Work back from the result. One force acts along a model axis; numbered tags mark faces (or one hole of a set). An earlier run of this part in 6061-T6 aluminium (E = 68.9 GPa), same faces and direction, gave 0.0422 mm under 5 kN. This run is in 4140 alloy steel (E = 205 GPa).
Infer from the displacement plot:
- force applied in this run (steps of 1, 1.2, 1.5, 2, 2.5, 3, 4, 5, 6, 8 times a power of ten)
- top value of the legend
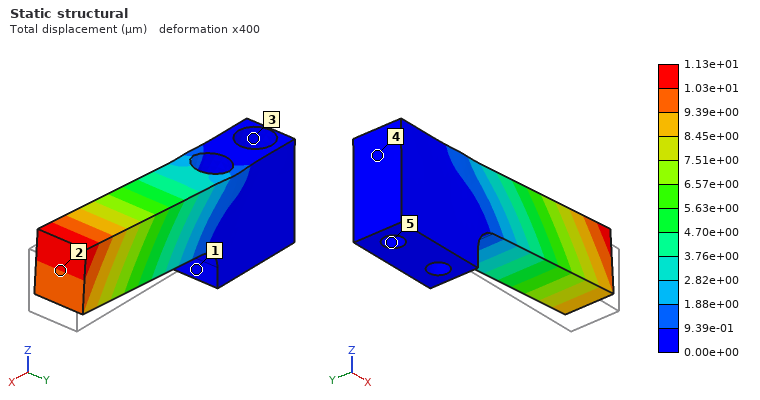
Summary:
4 kN
1.13e+01 µm
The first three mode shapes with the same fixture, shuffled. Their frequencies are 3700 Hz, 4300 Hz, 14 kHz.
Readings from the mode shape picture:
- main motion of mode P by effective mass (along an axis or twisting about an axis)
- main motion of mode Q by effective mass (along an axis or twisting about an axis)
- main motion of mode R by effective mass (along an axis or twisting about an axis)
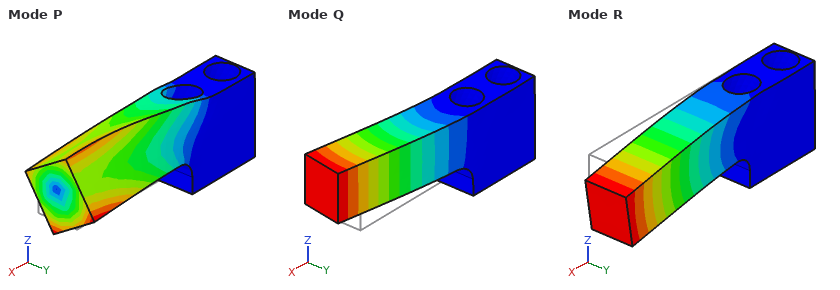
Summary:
twisting about X
along Y
along Z
